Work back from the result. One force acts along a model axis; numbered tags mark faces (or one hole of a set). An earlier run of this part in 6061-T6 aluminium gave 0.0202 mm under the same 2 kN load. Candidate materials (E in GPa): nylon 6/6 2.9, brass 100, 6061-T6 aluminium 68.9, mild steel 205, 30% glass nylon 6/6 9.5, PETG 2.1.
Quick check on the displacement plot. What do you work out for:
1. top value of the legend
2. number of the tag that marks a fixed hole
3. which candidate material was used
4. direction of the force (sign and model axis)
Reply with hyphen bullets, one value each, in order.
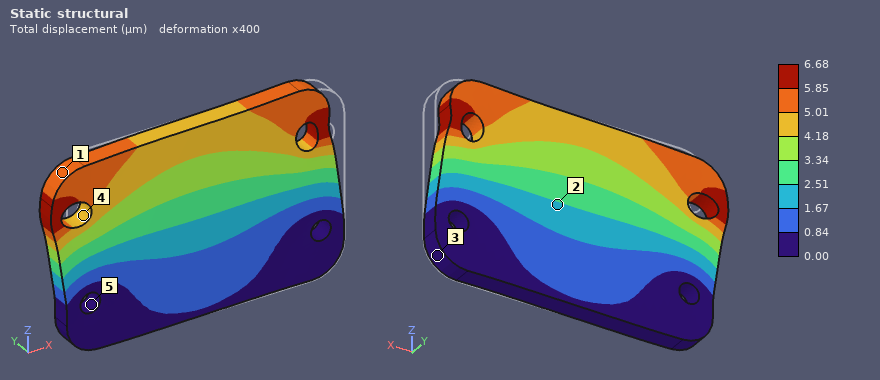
- 6.68 µm
- 5
- mild steel
- -X
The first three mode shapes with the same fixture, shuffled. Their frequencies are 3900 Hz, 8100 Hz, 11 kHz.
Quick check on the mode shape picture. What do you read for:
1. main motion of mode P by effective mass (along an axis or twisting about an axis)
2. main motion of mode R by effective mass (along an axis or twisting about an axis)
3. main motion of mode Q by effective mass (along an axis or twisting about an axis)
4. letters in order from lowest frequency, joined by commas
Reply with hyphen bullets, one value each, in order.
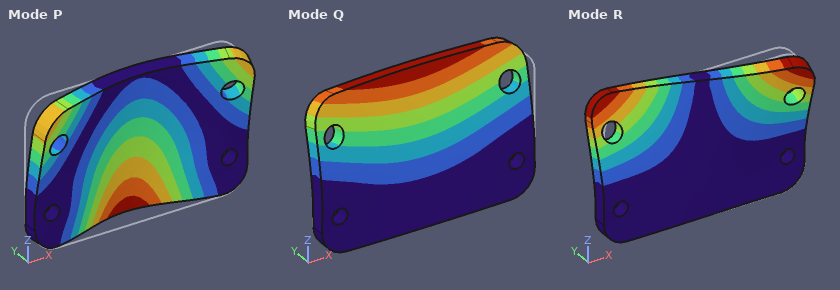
- along Y
- twisting about Z
- along Y
- Q, R, P
